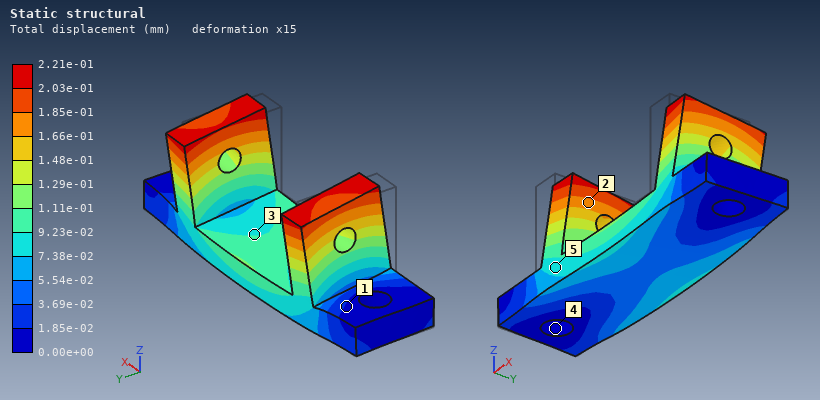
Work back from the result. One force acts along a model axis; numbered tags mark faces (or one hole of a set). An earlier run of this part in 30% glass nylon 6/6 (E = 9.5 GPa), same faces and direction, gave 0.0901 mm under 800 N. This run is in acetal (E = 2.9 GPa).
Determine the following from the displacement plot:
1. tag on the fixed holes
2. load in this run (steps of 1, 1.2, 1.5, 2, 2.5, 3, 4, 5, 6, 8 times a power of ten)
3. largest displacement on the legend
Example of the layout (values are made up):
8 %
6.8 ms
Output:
4
600 N
2.21e-01 mm
